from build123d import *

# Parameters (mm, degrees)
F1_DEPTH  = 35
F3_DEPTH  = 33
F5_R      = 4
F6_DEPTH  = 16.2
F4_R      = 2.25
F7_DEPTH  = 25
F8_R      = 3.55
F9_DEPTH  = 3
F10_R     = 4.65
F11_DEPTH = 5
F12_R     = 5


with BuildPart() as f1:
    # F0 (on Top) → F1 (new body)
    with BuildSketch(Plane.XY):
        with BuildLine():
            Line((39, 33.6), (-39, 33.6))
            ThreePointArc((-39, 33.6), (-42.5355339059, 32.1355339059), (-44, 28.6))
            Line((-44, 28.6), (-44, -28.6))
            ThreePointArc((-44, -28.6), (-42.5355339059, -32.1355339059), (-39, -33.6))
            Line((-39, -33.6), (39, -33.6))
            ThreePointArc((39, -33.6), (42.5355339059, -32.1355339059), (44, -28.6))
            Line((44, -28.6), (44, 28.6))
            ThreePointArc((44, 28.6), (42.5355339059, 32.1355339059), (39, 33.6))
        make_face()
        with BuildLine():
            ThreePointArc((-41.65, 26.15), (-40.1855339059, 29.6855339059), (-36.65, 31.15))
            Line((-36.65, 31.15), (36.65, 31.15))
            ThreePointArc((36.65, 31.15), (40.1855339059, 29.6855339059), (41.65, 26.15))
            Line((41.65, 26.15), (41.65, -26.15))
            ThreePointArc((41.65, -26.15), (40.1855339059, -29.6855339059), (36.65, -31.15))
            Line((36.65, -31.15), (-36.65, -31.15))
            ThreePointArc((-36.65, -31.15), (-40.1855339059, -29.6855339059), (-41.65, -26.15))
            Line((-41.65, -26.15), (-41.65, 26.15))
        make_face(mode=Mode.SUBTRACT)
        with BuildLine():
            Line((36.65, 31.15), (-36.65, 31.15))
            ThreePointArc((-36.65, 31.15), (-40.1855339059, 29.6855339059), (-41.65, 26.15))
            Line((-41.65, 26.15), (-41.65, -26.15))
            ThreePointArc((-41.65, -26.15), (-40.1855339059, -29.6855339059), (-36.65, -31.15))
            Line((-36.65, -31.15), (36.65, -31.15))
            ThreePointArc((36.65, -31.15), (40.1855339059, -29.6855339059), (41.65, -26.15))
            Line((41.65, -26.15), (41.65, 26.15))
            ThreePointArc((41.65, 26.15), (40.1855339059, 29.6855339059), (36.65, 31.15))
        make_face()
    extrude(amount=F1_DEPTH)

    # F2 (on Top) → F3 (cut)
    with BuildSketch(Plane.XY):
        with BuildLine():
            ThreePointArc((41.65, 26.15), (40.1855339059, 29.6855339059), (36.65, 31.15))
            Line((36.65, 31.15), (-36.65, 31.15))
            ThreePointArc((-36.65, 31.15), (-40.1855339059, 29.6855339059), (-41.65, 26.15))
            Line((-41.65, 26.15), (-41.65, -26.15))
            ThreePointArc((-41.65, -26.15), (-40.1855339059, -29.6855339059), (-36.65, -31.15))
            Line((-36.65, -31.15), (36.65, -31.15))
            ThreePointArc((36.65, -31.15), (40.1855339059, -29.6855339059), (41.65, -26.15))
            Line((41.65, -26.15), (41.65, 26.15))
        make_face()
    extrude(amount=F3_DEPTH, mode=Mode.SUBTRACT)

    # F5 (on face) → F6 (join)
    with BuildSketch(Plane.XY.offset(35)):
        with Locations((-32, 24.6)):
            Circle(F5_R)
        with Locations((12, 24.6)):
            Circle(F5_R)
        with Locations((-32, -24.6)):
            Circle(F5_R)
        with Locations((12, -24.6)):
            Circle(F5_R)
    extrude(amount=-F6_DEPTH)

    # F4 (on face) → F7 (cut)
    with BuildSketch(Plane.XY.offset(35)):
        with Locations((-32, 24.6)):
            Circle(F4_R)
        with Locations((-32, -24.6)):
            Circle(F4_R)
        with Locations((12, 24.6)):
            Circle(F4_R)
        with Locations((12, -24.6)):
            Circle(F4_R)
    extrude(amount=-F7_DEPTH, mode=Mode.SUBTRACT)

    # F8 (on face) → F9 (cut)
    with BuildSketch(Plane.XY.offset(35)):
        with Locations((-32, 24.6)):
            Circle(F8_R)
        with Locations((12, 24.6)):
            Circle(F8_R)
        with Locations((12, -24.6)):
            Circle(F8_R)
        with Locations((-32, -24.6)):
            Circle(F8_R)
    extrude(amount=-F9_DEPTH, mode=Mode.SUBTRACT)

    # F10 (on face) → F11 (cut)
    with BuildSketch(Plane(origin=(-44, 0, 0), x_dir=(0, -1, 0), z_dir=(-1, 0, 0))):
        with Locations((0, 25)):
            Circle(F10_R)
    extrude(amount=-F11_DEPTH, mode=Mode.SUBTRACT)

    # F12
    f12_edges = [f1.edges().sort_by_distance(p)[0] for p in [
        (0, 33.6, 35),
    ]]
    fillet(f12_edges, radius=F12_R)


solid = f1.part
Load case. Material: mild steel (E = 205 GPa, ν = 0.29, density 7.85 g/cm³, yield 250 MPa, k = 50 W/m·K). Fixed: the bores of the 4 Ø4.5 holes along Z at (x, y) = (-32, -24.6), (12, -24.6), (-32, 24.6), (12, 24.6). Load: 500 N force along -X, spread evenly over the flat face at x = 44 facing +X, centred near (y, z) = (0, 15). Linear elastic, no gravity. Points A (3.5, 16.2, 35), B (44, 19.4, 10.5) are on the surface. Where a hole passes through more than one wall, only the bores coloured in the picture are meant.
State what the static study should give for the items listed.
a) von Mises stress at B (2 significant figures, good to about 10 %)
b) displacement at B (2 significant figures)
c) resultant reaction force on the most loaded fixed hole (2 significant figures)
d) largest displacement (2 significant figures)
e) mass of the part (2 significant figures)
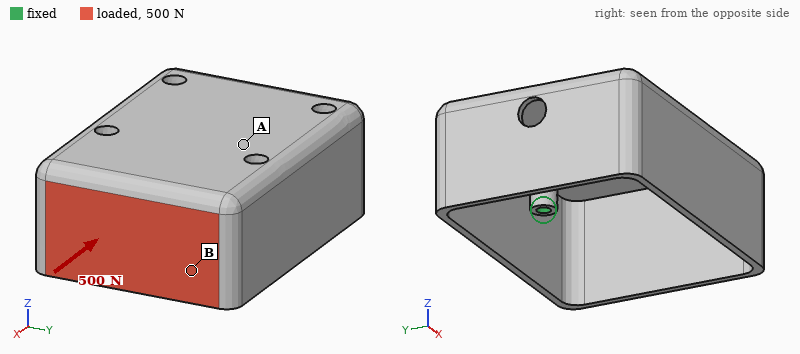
29 MPa
31 µm
160 N
78 µm
280 g
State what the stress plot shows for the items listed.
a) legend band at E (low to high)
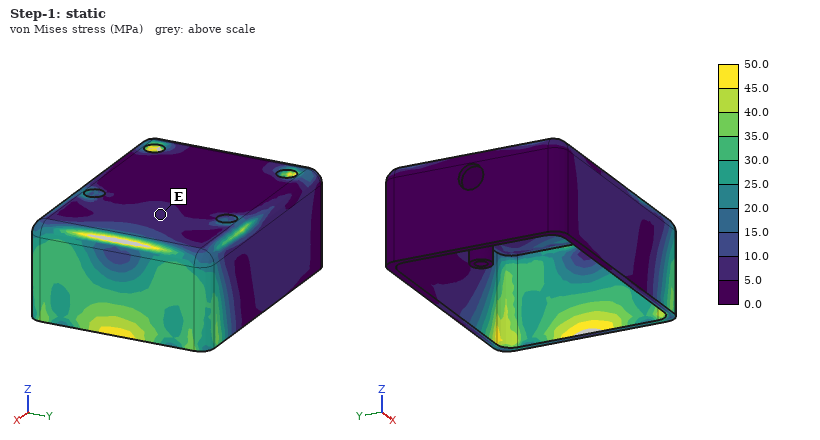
5.0 to 10.0 MPa
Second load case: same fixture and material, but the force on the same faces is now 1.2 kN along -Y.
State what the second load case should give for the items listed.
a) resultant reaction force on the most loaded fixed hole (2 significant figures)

1.0 kN
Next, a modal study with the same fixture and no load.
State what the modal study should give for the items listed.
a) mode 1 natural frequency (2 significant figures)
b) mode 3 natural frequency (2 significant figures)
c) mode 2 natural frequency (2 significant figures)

1900 Hz
2400 Hz
2000 Hz
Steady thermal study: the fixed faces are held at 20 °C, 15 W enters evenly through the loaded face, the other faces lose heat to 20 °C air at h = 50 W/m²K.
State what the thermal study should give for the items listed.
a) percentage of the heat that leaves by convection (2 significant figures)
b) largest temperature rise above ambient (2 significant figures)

80 %
41 K
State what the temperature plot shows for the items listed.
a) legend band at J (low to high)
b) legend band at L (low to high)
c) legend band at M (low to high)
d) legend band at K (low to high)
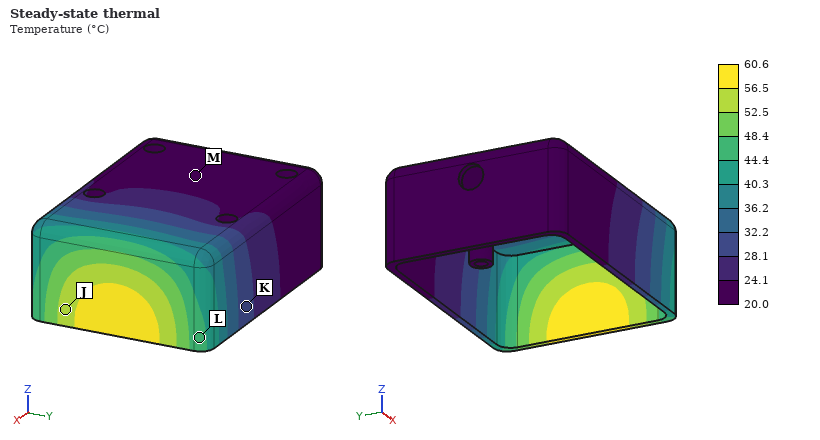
52.5 to 56.5 °C
44.4 to 48.4 °C
20.0 to 24.1 °C
28.1 to 32.2 °C
